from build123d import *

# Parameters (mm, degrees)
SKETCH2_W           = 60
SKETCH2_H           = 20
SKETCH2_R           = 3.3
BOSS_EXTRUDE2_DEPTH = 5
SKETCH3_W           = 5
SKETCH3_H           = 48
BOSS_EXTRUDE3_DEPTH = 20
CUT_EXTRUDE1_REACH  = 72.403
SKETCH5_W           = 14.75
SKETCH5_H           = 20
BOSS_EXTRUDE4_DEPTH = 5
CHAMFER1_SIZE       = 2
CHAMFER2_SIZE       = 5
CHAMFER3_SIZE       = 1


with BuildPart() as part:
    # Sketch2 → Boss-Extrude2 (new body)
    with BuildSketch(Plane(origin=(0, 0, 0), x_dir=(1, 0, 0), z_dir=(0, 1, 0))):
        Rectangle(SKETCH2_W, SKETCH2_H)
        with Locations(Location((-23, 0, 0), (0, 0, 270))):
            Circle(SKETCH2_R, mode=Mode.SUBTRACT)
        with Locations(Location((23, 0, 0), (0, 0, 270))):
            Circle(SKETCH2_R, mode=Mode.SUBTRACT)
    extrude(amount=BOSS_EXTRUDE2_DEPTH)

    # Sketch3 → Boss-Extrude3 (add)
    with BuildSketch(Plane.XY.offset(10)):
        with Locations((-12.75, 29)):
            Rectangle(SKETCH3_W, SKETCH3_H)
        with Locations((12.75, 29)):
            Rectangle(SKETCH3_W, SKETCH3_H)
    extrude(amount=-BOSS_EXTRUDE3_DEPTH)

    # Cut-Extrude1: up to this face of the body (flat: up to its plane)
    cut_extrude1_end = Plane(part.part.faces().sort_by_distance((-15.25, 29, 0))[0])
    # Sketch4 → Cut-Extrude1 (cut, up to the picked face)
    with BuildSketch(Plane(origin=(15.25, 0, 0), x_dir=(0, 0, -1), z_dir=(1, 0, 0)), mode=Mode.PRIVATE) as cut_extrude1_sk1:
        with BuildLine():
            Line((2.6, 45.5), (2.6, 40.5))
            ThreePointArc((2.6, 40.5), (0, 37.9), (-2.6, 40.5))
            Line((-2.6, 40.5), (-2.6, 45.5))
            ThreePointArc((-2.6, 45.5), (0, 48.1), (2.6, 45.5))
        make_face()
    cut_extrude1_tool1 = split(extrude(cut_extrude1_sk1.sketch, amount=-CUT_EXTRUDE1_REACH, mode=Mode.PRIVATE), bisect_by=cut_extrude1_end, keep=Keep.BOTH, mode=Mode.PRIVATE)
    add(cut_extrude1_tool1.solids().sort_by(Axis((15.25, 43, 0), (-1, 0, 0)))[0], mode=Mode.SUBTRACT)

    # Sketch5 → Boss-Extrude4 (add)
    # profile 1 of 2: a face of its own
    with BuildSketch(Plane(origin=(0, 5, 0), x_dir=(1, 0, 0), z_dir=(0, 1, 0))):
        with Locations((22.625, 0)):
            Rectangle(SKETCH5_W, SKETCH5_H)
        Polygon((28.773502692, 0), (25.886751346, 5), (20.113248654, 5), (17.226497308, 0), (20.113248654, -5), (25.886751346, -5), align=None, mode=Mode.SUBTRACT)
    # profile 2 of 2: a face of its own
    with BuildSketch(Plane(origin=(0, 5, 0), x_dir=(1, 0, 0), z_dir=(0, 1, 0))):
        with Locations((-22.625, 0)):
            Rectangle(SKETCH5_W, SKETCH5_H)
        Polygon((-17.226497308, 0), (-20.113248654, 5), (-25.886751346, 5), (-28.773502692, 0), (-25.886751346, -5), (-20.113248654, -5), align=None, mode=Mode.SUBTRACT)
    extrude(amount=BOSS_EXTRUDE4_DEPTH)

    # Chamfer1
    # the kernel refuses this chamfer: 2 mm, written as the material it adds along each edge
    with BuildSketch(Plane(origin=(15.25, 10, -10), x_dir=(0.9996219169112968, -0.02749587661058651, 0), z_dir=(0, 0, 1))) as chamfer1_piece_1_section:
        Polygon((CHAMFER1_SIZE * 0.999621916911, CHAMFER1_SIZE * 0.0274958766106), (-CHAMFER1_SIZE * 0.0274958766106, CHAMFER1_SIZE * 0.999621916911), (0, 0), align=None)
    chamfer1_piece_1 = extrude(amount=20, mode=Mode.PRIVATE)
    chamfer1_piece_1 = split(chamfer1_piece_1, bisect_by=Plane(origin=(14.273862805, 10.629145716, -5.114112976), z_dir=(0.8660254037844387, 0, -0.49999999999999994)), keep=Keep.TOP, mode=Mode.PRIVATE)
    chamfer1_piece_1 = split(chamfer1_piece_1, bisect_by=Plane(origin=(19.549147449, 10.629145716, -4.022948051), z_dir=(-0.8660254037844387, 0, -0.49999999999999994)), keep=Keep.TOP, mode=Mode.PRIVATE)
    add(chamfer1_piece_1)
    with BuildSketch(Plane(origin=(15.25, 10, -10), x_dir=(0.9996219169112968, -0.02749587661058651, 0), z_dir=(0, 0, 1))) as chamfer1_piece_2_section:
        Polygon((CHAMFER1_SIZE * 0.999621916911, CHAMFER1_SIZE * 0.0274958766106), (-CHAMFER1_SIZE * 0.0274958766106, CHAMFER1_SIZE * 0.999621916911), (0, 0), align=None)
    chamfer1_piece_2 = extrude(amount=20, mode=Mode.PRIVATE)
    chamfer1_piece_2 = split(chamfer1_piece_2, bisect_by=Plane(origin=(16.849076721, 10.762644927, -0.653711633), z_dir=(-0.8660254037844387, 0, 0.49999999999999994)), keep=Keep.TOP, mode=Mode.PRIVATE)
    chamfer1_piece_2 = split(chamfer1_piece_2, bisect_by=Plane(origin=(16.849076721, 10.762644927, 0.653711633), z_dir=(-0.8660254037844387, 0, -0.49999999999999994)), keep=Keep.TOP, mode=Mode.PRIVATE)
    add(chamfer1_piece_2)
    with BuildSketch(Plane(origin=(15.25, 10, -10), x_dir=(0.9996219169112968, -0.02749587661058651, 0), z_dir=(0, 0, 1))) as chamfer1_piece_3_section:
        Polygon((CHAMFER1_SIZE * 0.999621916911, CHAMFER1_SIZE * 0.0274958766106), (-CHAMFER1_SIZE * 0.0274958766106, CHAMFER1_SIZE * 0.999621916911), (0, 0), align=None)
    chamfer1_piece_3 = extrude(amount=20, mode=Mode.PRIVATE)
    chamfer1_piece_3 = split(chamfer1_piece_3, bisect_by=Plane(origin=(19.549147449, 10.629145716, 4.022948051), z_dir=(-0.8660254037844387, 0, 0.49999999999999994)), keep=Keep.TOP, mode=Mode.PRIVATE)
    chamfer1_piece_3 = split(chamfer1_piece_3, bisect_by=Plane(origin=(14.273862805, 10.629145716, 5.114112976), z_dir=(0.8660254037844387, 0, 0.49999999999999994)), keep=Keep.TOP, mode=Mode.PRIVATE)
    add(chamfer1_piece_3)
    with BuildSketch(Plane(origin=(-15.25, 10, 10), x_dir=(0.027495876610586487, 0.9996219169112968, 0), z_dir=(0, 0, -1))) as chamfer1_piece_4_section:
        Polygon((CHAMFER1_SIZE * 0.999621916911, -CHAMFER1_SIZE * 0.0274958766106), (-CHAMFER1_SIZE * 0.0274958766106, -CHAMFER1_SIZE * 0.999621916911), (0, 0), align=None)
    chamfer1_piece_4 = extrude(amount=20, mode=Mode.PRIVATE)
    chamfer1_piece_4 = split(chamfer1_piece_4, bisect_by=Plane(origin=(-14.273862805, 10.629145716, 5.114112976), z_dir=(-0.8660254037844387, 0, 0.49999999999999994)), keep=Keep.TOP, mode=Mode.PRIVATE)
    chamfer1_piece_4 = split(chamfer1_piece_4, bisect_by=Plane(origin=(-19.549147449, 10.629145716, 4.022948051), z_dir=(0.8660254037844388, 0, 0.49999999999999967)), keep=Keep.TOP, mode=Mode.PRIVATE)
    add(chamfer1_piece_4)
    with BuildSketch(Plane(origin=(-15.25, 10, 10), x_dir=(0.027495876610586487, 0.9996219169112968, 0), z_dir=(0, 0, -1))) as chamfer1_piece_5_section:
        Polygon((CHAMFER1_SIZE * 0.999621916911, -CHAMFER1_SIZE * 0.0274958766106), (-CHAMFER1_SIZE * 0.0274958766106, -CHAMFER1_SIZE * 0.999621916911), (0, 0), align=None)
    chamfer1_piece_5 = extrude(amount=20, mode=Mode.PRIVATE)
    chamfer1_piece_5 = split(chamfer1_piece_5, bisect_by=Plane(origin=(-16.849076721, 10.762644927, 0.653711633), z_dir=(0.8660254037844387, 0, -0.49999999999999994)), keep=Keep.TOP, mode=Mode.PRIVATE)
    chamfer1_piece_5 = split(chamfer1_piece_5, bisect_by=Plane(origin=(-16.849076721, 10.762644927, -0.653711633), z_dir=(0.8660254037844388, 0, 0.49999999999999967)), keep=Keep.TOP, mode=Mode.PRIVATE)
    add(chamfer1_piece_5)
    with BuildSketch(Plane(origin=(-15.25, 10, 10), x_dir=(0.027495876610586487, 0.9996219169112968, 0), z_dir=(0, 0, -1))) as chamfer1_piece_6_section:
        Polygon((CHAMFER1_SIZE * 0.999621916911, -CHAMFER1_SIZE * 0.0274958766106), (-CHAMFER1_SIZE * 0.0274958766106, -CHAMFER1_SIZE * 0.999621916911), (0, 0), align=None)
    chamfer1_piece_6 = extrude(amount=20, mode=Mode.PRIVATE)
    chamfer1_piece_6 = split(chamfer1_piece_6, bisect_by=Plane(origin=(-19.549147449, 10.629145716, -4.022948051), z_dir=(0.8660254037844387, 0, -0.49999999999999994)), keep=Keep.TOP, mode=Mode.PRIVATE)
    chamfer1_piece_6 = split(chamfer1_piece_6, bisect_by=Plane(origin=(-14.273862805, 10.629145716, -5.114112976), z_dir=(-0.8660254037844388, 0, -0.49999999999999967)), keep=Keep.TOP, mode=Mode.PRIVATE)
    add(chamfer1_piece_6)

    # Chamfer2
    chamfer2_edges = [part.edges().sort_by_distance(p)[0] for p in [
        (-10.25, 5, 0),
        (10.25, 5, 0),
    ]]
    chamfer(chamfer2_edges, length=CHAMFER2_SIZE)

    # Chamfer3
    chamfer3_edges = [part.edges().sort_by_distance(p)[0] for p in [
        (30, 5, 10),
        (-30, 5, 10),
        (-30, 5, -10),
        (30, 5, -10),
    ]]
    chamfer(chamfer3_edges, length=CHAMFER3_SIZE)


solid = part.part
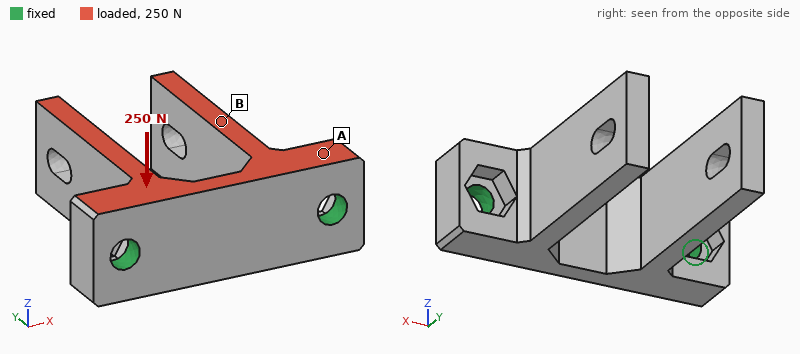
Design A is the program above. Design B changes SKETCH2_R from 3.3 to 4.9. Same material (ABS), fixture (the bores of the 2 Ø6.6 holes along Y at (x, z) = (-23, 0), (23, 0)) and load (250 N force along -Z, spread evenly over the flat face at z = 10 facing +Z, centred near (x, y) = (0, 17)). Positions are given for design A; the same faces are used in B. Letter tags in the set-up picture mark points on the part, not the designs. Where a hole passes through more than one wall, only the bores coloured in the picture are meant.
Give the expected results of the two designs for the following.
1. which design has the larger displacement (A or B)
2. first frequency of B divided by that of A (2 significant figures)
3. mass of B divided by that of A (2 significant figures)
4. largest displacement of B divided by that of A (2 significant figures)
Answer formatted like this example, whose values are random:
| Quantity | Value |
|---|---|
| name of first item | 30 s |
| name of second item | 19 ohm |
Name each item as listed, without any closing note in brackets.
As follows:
| Quantity | Value |
|---|---|
| which design has the larger displacement | A |
| first frequency of B divided by that of A | 1.0 |
| mass of B divided by that of A | 0.98 |
| largest displacement of B divided by that of A | 0.67 |
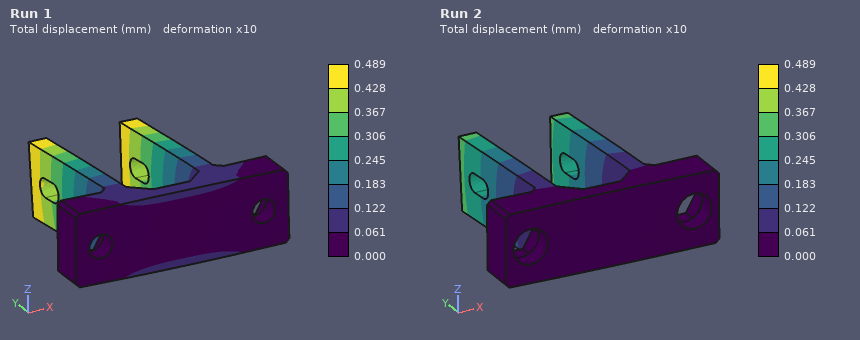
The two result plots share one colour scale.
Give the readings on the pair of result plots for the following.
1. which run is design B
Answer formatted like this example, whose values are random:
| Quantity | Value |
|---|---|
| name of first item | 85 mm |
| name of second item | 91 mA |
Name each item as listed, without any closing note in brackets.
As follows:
| Quantity | Value |
|---|---|
| which run is design B | Run 2 |
